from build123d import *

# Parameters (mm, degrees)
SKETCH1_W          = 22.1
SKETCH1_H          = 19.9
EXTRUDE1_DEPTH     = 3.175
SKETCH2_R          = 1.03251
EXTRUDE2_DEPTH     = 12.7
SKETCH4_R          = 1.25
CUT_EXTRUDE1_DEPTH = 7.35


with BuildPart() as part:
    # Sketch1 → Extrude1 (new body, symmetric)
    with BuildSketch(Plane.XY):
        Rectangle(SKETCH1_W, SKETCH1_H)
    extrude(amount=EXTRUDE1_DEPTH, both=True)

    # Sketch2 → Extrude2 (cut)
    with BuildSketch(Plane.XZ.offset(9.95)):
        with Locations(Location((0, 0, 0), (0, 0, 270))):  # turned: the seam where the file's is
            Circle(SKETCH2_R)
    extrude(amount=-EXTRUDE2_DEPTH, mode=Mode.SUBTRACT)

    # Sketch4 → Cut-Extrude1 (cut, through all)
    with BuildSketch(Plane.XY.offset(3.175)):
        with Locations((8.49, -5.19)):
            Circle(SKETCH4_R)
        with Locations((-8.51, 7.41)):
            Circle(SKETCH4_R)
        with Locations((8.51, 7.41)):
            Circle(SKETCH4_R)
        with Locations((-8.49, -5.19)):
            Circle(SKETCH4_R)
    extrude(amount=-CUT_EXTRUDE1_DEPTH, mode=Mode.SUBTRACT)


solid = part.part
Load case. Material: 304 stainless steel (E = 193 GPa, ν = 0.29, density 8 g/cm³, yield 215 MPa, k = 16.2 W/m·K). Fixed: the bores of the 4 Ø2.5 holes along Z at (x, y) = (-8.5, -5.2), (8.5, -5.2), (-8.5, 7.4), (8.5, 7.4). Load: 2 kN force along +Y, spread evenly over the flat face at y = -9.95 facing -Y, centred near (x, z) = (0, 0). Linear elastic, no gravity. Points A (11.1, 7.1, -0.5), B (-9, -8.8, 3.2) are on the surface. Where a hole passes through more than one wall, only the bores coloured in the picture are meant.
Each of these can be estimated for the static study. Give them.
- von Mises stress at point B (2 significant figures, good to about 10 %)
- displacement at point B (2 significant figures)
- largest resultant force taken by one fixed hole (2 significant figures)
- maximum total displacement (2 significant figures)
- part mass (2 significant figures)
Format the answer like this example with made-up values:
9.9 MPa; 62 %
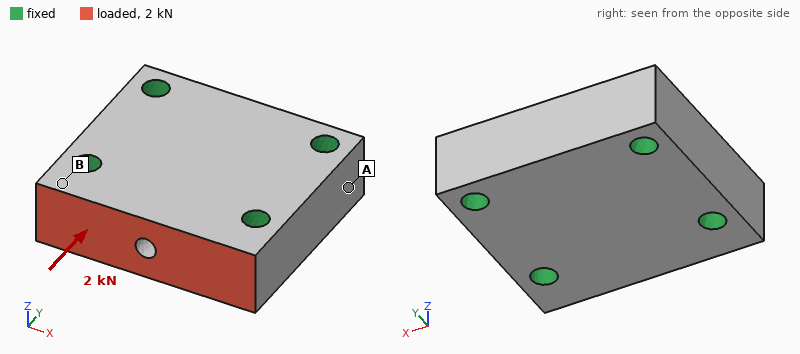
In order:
17 MPa; 0.25 µm; 810 N; 0.91 µm; 21 g
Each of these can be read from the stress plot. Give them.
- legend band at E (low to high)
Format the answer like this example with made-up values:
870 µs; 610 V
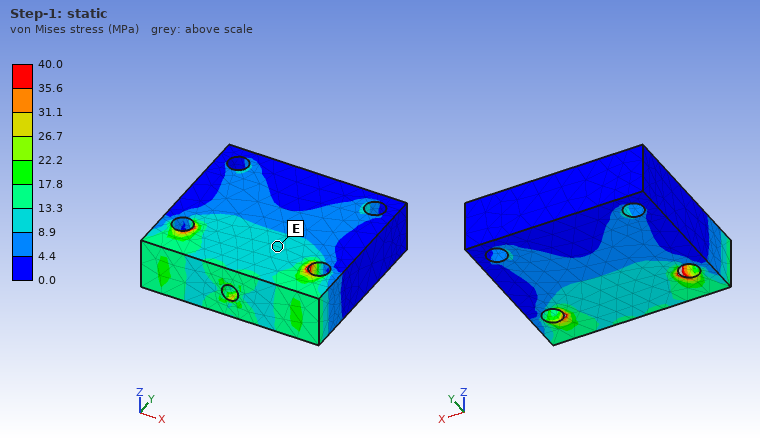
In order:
8.9 to 13.3 MPa
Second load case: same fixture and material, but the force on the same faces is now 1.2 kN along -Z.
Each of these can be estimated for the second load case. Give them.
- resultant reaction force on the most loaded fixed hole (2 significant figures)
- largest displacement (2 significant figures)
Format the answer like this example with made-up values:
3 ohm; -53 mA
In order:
650 N; 2.7 µm
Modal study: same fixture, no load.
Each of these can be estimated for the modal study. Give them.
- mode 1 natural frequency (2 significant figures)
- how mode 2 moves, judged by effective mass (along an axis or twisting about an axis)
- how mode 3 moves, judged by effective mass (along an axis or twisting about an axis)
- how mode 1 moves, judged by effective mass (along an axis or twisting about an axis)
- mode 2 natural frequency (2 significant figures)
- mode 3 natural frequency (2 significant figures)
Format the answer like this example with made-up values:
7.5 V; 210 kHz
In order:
63 kHz; twisting about X; along Y; along Z; 73 kHz; 82 kHz
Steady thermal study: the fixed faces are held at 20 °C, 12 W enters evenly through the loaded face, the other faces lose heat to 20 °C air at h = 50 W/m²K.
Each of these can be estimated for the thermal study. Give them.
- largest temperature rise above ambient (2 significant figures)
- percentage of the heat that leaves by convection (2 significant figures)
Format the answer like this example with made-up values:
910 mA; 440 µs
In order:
37 K; 3.5 %
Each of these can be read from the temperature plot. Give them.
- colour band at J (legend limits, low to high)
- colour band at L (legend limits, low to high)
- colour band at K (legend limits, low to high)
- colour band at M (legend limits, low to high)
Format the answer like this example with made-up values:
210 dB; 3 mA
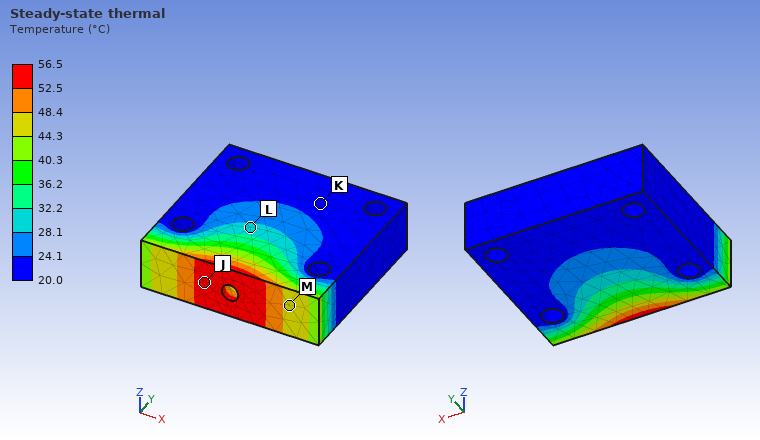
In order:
52.5 to 56.5 °C; 28.1 to 32.2 °C; 20.0 to 24.1 °C; 44.3 to 48.4 °C
